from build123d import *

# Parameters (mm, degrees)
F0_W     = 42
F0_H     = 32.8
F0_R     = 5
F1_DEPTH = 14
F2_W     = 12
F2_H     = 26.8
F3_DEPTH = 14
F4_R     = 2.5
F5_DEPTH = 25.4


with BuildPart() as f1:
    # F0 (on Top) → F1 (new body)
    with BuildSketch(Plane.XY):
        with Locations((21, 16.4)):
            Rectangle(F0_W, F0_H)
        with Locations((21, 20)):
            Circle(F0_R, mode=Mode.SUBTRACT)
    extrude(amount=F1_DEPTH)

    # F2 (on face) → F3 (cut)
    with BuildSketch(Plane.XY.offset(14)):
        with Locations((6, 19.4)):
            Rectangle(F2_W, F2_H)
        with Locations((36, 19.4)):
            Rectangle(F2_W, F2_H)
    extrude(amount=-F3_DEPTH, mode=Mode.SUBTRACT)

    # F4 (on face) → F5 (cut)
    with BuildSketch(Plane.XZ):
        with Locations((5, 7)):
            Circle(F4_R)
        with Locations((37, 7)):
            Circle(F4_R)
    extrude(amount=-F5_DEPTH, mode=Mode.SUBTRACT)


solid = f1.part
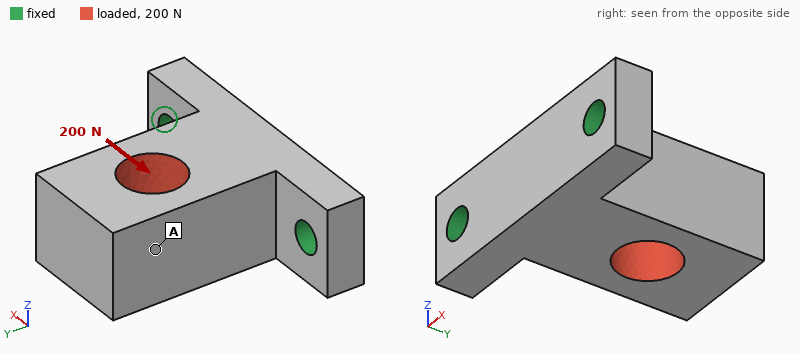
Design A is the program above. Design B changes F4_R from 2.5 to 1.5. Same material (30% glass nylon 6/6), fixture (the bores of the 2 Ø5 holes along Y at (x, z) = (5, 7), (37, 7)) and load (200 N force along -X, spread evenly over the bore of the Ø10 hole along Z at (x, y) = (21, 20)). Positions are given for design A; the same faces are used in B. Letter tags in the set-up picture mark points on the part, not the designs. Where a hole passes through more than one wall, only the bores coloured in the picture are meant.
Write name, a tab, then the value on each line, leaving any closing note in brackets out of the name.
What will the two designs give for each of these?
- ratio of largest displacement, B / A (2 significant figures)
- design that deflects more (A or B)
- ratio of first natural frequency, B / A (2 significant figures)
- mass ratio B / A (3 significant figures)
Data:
ratio of largest displacement, B / A	1.1
design that deflects more	B
ratio of first natural frequency, B / A	0.89
mass ratio B / A	1.02
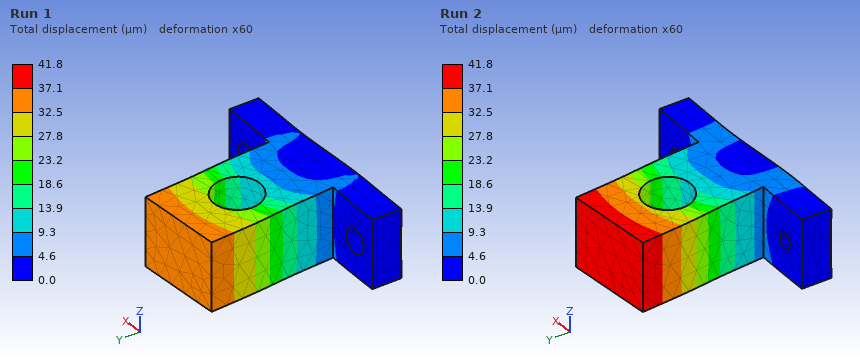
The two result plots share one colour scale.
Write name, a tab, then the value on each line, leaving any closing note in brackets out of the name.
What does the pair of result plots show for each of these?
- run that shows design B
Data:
run that shows design B	Run 2
